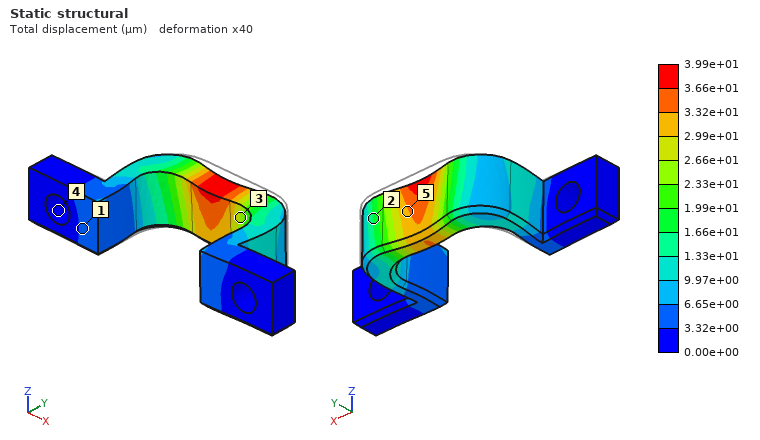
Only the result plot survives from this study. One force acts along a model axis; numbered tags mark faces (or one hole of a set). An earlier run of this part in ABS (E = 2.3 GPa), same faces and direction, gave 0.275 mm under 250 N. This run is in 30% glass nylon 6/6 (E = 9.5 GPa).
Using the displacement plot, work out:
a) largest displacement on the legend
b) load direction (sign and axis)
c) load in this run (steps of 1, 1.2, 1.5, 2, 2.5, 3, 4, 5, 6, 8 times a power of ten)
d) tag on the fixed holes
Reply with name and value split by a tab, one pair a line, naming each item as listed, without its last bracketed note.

largest displacement on the legend	3.99e+01 µm
load direction	-Y
load in this run	150 N
tag on the fixed holes	4
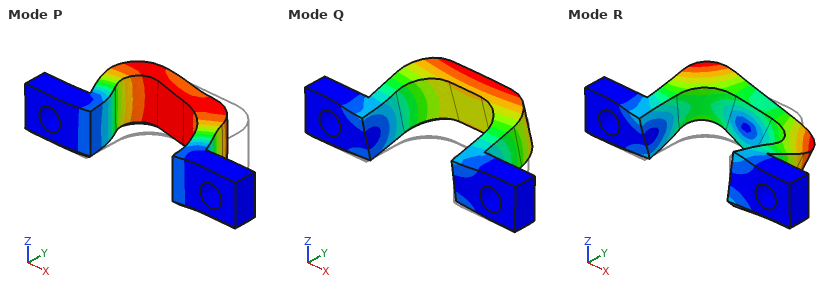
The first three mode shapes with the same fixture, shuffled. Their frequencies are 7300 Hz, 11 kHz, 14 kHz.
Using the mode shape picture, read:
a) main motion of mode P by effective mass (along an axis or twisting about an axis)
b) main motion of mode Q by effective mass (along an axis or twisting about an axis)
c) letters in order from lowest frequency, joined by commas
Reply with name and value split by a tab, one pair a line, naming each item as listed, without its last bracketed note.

main motion of mode P by effective mass	along X
main motion of mode Q by effective mass	along Z
letters in order from lowest frequency, joined by commas	Q, P, R
